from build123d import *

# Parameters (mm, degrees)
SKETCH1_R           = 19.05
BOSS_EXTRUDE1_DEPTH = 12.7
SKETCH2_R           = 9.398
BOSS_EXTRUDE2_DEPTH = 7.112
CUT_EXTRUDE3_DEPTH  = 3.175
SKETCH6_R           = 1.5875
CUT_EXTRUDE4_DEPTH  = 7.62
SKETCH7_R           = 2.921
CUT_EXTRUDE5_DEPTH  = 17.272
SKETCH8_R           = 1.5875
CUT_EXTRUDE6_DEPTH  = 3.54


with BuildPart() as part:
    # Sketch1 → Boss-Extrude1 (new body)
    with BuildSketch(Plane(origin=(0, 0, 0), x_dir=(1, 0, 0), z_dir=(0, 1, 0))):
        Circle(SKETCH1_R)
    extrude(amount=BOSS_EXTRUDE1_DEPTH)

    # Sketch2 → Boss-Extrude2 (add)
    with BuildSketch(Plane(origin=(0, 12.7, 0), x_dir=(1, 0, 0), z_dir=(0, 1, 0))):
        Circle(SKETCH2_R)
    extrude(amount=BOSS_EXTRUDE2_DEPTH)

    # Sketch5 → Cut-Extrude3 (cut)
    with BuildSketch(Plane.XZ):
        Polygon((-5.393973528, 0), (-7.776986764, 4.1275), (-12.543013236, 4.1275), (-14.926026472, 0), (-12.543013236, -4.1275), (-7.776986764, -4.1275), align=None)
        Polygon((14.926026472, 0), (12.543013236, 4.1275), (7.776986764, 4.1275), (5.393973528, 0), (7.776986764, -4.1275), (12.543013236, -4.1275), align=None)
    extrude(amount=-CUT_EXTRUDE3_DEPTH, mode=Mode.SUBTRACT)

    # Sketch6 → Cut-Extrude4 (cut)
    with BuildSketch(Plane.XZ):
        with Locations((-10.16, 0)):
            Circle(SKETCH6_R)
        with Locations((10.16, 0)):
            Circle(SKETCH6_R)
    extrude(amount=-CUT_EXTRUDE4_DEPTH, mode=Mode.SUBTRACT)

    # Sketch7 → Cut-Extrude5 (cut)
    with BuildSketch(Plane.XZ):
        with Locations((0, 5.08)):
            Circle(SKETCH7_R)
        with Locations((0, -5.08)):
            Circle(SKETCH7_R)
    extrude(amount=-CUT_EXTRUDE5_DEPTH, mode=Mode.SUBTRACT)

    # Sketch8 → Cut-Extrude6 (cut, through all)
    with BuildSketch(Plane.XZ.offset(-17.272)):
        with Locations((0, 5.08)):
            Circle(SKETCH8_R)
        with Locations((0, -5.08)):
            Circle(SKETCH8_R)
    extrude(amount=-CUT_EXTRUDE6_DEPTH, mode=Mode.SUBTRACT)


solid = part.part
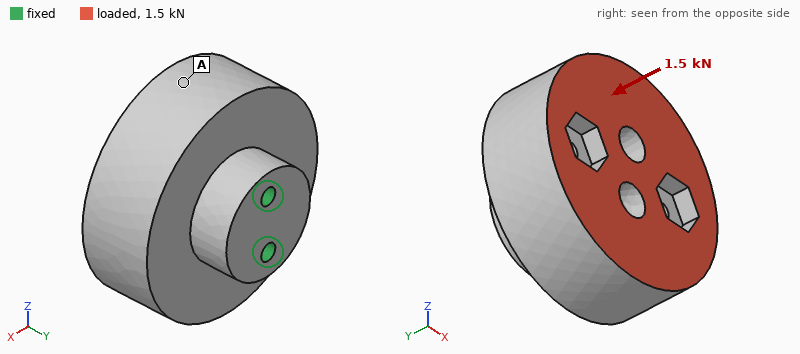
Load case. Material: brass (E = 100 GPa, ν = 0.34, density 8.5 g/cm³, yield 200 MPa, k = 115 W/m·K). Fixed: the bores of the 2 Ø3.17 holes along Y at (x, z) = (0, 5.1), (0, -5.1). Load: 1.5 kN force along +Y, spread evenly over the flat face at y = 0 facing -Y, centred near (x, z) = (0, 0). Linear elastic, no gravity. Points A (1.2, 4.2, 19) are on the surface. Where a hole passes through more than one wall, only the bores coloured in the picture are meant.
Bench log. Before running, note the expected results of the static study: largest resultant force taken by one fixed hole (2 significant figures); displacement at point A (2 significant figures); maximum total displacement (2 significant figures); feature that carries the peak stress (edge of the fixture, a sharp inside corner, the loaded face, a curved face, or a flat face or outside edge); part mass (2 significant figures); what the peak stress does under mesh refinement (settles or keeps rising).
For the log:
750 N
3.1 µm
3.2 µm
edge of the fixture
130 g
keeps rising
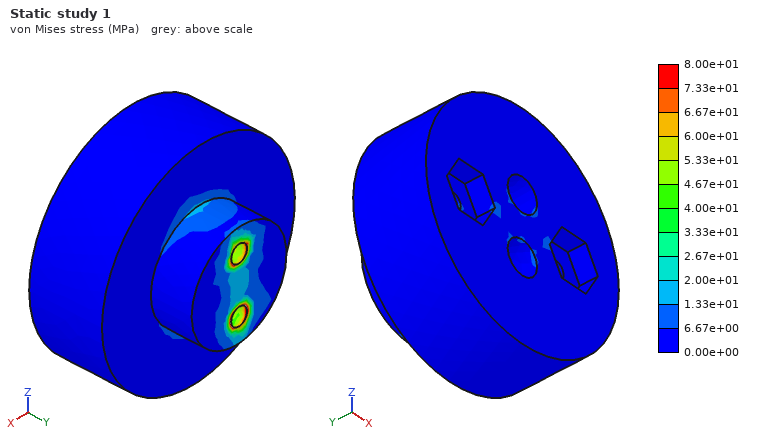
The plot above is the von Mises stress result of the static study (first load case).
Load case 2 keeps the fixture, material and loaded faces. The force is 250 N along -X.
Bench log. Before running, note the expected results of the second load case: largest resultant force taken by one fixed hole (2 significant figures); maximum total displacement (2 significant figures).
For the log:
130 N
31 µm
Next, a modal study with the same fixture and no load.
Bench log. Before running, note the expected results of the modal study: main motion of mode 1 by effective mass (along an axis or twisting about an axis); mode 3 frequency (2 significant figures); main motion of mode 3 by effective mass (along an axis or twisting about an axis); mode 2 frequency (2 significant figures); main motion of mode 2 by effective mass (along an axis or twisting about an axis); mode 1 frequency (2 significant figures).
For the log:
along X
5200 Hz
twisting about Y
4100 Hz
along Z
1900 Hz
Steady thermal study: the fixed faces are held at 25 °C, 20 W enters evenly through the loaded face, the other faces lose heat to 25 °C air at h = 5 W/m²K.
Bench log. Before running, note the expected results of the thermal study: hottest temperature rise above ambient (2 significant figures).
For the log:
14 K
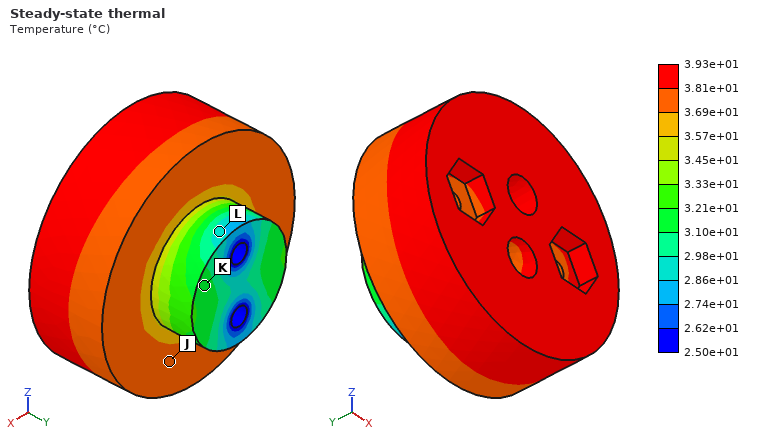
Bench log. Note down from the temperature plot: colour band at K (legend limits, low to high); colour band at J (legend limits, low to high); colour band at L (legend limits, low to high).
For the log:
3.10e+01 to 3.21e+01 °C
3.69e+01 to 3.81e+01 °C
2.86e+01 to 2.98e+01 °C
